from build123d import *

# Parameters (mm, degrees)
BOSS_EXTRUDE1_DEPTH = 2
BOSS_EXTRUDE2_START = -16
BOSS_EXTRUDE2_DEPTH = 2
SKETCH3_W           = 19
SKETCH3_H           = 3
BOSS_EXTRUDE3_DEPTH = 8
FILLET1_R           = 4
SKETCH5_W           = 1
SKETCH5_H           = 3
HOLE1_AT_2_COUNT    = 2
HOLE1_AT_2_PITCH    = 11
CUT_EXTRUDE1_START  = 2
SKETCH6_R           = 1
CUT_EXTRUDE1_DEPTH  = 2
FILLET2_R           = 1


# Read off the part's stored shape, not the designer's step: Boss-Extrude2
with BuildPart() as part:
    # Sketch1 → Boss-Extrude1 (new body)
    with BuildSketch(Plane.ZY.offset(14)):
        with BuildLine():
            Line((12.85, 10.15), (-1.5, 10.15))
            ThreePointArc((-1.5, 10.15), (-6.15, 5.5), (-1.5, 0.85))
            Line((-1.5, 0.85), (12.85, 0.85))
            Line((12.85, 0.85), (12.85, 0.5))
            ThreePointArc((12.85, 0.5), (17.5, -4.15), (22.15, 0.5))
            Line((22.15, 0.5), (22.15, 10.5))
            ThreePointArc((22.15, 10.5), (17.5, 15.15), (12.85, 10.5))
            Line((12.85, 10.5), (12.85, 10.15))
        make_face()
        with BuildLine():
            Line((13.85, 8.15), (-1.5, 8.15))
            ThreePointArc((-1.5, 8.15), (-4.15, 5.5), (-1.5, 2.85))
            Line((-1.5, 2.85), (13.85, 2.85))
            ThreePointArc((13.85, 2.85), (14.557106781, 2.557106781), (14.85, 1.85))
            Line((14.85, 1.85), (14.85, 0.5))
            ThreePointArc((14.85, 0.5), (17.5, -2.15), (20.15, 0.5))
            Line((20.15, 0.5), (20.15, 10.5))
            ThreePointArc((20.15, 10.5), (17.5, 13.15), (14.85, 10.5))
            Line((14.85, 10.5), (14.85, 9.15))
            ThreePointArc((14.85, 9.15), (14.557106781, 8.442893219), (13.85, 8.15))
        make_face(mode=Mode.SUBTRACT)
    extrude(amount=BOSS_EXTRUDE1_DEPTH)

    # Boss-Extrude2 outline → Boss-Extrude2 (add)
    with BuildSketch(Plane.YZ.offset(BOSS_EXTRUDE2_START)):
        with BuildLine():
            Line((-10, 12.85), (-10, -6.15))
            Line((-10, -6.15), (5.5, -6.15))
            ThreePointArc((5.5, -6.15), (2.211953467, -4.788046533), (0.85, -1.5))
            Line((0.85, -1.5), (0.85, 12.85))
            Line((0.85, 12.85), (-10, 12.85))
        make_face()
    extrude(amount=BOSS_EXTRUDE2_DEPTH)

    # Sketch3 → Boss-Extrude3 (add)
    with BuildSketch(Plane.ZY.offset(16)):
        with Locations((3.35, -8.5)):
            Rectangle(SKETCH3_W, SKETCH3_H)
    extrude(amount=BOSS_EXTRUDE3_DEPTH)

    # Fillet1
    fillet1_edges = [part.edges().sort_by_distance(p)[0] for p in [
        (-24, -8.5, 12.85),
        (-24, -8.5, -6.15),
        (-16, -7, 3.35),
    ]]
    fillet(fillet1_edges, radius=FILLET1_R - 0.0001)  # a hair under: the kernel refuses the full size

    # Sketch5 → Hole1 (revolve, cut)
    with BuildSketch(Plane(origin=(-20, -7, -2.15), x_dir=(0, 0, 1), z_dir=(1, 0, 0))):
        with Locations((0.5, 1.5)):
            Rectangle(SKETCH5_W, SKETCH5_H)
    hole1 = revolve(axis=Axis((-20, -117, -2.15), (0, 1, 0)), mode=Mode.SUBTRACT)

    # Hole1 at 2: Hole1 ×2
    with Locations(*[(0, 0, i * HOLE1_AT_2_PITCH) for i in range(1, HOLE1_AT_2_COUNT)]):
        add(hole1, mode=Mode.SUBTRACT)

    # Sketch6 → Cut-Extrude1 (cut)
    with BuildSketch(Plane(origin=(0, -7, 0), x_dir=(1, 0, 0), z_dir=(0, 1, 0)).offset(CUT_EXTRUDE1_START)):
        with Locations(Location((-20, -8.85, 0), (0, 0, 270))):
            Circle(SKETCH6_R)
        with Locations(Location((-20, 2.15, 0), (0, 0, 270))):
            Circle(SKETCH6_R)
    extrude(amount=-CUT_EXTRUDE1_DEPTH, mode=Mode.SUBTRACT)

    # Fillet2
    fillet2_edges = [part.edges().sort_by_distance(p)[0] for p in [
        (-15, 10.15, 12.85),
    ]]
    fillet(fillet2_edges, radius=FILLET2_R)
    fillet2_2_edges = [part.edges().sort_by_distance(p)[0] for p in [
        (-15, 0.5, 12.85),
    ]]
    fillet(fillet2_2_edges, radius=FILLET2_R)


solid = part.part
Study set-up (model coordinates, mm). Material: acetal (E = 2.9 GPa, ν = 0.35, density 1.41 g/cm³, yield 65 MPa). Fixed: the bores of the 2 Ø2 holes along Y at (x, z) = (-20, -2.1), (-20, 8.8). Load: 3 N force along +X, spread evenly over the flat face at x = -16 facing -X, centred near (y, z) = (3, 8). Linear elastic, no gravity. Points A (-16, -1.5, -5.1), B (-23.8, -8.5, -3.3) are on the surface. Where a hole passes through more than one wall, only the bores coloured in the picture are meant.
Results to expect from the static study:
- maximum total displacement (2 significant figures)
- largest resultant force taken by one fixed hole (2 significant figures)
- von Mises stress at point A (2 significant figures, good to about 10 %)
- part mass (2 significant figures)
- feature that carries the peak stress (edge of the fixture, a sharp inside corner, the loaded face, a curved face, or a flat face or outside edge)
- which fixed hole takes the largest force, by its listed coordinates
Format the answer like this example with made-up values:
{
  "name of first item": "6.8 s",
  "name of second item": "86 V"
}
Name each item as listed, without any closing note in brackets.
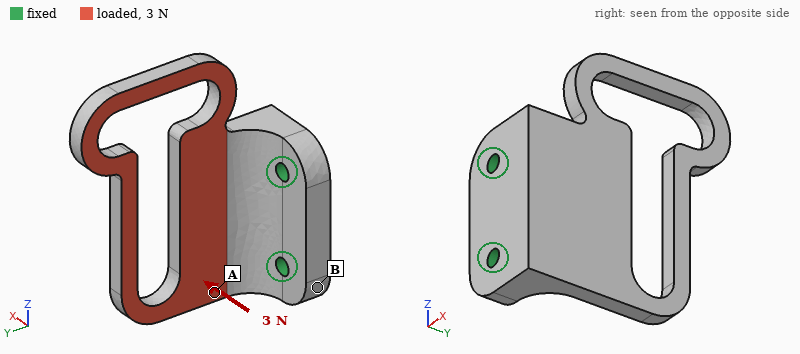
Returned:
{
  "maximum total displacement": "0.46 mm",
  "largest resultant force taken by one fixed hole": "2.6 N",
  "von Mises stress at point A": "1.5 MPa",
  "part mass": "1.7 g",
  "feature that carries the peak stress": "a curved face",
  "which fixed hole takes the largest force, by its listed coordinates": "(-20, 8.8)"
}
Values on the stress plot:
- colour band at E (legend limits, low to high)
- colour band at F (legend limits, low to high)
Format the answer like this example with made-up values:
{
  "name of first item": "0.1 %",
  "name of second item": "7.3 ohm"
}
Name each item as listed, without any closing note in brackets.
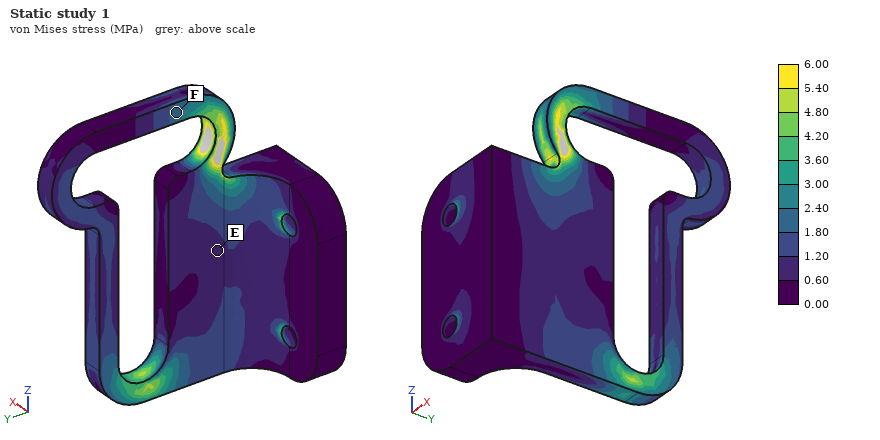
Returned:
{
  "colour band at E": "0.60 to 1.20 MPa",
  "colour band at F": "1.80 to 2.40 MPa"
}
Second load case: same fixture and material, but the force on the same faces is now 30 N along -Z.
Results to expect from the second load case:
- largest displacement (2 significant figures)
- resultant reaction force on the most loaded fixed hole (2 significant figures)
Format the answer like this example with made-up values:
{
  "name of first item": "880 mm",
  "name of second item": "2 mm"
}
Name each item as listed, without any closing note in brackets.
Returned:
{
  "largest displacement": "0.40 mm",
  "resultant reaction force on the most loaded fixed hole": "32 N"
}
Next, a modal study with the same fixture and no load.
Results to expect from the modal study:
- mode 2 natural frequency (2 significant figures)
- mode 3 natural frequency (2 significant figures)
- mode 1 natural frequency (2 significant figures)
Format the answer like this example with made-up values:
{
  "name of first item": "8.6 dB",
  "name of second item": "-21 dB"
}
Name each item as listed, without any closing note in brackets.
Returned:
{
  "mode 2 natural frequency": "1900 Hz",
  "mode 3 natural frequency": "1900 Hz",
  "mode 1 natural frequency": "630 Hz"
}
